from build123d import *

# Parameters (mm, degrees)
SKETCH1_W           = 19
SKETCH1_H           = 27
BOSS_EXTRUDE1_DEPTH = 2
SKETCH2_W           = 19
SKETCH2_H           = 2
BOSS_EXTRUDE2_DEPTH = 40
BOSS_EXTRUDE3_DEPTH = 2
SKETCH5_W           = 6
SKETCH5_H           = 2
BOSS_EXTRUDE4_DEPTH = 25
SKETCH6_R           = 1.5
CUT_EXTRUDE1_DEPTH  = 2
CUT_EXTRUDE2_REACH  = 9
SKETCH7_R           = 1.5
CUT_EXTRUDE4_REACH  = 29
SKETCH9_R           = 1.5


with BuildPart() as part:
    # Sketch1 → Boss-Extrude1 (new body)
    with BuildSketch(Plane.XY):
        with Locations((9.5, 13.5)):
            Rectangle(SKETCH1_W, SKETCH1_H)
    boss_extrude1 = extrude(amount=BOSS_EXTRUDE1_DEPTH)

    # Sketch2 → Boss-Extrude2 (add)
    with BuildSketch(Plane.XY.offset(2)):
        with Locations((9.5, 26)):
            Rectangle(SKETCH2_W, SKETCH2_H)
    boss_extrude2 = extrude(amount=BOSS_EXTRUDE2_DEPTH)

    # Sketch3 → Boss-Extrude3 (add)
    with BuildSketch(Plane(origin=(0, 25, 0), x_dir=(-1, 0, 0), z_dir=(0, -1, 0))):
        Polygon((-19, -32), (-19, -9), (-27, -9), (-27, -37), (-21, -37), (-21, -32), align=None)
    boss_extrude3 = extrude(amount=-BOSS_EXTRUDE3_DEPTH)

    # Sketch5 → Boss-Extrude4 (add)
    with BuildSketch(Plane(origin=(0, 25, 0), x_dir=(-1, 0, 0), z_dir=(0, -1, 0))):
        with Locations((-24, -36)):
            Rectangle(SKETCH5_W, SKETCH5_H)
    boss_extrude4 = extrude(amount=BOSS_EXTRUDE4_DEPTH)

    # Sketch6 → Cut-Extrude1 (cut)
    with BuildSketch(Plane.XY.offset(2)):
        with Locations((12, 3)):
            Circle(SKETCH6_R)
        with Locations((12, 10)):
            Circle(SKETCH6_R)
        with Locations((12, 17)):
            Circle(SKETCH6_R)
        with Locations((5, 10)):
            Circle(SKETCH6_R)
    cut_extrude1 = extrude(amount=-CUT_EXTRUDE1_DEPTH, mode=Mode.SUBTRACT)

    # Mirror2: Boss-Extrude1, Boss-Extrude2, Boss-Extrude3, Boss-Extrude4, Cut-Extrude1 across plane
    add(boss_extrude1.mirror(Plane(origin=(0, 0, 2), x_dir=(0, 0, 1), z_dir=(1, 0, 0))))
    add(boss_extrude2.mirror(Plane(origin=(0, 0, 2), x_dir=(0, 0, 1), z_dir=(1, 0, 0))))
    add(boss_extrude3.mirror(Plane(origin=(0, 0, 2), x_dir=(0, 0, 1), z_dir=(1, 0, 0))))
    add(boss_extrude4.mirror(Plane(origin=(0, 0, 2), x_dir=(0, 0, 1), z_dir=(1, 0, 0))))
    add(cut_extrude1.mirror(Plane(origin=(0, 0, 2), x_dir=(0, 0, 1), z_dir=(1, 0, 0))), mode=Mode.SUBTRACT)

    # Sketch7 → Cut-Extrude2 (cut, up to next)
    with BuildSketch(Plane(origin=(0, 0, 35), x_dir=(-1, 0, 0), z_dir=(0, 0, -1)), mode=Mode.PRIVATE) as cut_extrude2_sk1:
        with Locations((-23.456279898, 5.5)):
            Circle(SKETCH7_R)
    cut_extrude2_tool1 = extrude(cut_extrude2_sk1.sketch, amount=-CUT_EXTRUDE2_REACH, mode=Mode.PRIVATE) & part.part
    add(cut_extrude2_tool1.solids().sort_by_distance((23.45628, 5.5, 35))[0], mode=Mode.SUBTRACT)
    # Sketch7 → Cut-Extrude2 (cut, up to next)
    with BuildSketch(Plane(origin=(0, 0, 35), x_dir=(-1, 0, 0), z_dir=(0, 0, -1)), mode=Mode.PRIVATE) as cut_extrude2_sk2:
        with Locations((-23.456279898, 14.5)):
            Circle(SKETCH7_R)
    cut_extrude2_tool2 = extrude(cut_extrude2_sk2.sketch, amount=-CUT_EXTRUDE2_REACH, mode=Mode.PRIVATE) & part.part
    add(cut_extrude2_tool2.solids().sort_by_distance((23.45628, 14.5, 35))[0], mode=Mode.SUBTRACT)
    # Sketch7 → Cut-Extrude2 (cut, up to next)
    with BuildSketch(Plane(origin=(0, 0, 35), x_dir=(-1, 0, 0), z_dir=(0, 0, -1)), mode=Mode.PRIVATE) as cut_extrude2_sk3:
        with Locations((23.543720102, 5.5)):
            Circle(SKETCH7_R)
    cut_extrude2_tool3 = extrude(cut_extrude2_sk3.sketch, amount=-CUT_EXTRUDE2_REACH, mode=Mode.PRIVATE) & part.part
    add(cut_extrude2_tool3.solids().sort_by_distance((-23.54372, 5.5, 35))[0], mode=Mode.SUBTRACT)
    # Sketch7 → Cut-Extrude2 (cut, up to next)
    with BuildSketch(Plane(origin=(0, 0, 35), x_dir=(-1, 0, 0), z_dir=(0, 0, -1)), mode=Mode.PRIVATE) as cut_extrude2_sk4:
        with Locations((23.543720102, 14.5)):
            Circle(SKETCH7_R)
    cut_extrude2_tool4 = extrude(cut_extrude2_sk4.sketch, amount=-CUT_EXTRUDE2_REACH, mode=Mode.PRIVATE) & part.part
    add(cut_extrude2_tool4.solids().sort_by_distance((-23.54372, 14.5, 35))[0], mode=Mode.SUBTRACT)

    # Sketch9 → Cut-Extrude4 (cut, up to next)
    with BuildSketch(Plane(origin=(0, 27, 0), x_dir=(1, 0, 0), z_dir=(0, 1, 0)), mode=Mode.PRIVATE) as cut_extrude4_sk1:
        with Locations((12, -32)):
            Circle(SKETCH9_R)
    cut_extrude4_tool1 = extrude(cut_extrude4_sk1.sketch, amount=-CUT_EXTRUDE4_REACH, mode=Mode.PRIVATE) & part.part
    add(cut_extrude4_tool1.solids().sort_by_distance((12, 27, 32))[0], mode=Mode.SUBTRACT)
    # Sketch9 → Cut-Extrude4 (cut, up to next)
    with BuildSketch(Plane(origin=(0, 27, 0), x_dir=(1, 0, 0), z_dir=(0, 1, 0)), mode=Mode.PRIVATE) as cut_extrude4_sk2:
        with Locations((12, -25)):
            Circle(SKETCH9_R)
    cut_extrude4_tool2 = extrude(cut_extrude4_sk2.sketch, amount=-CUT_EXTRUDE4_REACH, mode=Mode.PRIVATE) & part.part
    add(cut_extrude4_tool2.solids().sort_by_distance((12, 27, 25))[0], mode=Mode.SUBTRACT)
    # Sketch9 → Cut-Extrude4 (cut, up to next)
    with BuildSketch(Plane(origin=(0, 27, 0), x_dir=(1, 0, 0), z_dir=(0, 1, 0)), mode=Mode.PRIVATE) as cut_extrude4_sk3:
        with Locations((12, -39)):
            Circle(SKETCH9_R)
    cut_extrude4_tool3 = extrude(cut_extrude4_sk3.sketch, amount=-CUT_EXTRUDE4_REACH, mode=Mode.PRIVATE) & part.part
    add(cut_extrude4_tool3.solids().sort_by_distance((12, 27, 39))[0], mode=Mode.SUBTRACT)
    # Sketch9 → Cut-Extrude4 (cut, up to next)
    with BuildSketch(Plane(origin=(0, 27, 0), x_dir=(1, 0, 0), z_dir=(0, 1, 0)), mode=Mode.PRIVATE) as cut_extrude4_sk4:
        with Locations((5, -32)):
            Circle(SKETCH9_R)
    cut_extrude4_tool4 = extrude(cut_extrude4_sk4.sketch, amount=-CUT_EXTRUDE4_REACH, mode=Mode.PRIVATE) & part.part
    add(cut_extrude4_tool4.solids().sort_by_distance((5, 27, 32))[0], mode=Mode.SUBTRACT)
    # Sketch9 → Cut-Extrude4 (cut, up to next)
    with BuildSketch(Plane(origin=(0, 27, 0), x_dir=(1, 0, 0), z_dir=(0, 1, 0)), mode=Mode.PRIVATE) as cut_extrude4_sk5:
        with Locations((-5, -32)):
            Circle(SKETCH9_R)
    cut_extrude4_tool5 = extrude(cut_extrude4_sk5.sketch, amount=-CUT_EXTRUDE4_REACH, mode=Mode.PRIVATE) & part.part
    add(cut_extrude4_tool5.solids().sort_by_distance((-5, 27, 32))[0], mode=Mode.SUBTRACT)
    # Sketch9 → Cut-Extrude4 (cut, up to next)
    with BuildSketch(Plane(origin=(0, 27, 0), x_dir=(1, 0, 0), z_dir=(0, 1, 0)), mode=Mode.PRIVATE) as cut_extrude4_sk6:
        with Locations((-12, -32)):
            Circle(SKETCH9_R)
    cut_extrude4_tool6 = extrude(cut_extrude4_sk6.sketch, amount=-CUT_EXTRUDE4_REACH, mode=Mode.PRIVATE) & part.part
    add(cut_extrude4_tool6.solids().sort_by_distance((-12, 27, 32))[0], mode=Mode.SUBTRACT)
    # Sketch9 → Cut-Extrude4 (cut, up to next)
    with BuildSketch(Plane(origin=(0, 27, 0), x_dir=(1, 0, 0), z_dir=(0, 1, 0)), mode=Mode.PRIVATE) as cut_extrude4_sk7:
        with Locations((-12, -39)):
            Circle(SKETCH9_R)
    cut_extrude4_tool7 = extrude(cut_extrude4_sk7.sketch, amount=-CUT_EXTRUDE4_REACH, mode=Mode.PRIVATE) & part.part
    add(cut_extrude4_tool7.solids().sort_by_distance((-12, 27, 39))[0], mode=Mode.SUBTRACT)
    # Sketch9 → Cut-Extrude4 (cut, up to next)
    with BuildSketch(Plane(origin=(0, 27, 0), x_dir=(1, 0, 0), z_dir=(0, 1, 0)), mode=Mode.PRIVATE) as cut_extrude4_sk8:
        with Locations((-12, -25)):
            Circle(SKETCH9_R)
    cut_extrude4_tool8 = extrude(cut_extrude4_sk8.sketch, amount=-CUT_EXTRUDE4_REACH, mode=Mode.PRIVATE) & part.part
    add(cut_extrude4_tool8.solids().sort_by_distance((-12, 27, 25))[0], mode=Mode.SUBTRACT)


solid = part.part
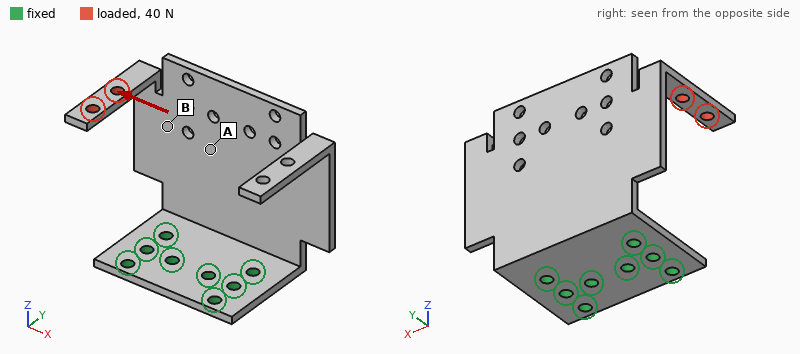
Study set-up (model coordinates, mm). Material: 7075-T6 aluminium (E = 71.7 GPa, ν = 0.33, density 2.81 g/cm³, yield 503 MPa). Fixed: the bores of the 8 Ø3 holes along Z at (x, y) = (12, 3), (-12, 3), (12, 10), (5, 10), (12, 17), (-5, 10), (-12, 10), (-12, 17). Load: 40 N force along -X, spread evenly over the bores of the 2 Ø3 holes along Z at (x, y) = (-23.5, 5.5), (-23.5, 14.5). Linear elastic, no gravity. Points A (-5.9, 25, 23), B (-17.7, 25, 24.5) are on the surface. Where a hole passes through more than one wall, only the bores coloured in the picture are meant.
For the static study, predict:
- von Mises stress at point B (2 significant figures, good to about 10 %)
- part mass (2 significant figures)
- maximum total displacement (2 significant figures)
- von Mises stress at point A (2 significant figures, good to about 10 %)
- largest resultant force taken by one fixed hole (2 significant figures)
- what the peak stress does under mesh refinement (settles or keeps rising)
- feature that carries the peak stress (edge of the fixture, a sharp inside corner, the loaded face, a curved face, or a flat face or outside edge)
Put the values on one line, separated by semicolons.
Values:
47 MPa; 18 g; 0.76 mm; 20 MPa; 70 N; keeps rising; a sharp inside corner
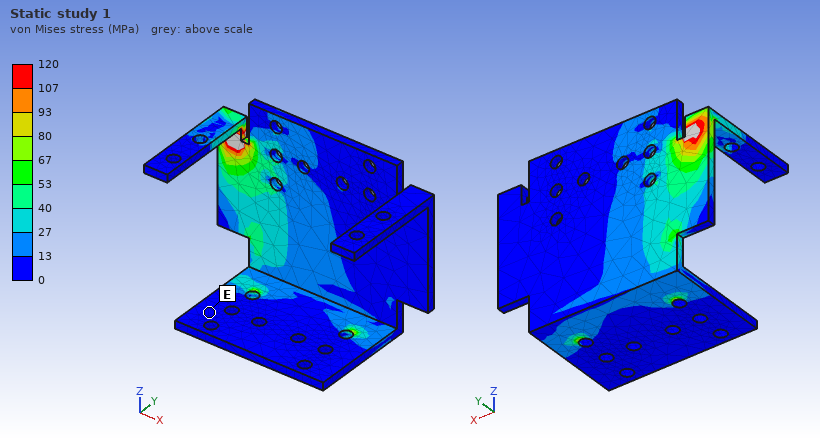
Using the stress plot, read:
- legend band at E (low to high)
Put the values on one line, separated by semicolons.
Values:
0 to 13 MPa
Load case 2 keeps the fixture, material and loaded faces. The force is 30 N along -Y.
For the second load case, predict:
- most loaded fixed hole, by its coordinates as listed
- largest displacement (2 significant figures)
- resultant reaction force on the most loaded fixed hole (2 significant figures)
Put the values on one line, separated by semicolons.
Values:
(-12, 17); 0.78 mm; 46 N
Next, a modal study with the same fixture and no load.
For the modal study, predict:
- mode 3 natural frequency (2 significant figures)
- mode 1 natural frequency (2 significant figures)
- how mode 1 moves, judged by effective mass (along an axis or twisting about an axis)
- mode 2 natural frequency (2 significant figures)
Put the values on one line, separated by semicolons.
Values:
1500 Hz; 590 Hz; along Y; 1000 Hz
